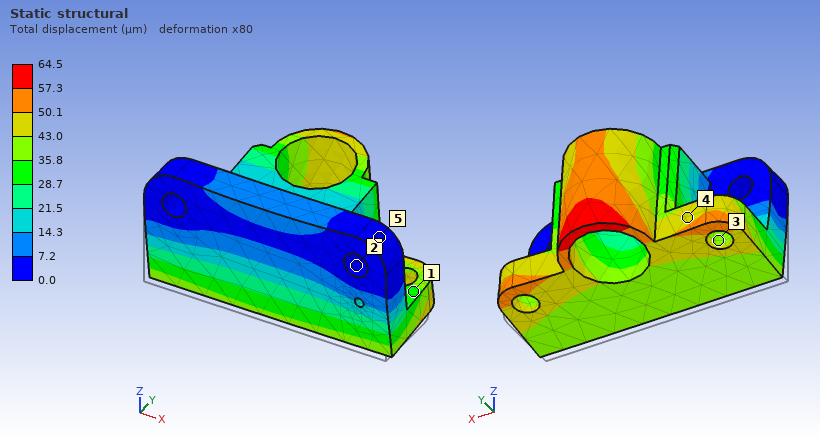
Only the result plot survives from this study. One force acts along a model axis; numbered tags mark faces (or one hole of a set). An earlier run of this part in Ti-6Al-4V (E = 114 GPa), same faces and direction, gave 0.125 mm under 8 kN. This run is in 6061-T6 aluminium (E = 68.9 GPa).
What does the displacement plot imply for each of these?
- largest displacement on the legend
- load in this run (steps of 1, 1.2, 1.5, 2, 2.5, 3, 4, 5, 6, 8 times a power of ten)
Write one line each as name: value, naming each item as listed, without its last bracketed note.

largest displacement on the legend: 64.5 µm
load in this run: 2.5 kN
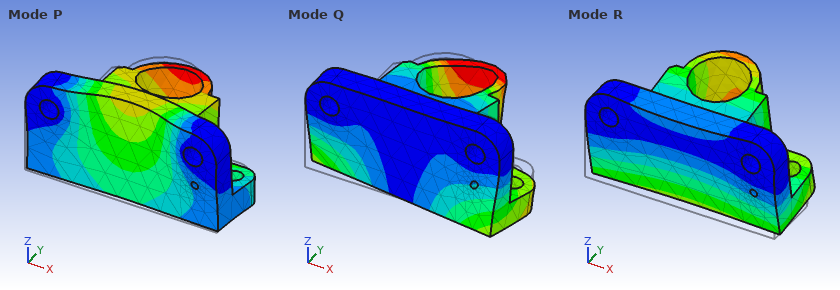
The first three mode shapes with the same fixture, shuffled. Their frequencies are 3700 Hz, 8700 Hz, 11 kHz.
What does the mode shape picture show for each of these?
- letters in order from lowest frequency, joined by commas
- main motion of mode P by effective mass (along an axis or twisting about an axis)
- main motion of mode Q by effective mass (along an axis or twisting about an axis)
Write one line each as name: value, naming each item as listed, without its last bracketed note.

letters in order from lowest frequency, joined by commas: R, Q, P
main motion of mode P by effective mass: along Y
main motion of mode Q by effective mass: along X
